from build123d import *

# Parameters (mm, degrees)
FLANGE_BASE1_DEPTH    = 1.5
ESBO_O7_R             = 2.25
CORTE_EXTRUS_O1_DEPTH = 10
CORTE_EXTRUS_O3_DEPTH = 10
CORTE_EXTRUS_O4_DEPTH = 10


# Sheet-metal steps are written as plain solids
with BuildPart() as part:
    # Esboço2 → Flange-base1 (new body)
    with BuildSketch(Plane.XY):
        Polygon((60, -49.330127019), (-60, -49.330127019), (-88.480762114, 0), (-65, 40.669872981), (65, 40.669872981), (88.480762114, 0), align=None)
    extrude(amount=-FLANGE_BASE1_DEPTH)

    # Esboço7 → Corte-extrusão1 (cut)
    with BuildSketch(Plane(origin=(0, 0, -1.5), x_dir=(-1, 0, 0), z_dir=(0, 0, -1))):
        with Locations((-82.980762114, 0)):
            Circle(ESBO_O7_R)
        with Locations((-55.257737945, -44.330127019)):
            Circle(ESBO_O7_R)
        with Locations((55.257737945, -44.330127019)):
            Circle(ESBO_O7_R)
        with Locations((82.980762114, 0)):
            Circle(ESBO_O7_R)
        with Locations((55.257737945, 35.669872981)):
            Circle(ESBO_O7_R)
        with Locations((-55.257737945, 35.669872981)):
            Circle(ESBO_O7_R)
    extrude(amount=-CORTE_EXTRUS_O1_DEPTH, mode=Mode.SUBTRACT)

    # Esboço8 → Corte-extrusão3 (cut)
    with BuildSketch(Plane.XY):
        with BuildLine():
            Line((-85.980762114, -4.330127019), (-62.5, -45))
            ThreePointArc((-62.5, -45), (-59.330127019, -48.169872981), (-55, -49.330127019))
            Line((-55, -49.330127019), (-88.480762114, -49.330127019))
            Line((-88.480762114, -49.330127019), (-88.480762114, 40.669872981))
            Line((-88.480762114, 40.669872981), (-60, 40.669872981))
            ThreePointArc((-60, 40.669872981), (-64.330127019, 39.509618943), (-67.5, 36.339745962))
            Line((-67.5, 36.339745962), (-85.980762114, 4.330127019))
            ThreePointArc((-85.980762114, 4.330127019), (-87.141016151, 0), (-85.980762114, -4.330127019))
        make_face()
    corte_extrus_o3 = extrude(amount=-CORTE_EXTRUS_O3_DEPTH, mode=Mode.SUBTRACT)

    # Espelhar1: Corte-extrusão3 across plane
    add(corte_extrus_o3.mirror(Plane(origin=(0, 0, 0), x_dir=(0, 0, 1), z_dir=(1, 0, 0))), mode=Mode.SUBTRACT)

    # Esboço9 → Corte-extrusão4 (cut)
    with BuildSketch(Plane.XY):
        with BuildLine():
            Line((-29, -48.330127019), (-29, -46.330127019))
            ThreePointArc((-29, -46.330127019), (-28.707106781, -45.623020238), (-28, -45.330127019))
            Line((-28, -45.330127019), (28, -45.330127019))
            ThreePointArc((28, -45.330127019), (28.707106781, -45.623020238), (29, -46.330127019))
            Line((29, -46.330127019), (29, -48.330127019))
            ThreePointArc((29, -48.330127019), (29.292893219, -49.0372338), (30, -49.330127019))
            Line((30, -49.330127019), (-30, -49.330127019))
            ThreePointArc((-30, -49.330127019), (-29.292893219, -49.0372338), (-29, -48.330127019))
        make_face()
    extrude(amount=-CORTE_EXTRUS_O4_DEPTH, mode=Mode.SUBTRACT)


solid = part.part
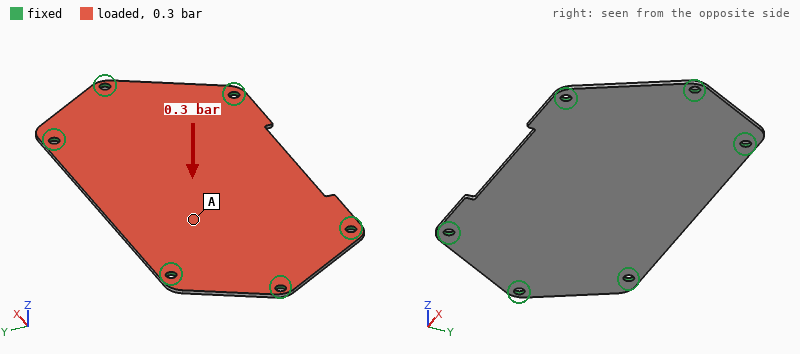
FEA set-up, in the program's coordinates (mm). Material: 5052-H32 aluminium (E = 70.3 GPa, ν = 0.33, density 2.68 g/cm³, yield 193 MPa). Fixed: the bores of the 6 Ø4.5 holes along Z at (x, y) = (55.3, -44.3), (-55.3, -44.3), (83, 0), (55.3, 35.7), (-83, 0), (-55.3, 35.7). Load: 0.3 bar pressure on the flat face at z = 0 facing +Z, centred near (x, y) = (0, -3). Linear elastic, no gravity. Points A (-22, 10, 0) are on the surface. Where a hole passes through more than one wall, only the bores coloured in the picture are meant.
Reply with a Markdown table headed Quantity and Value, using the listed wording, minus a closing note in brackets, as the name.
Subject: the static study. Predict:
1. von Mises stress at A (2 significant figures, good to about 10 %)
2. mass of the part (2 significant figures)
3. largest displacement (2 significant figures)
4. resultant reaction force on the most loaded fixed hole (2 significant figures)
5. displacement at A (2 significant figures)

| Quantity | Value |
|---|---|
| von Mises stress at A | 29 MPa |
| mass of the part | 53 g |
| largest displacement | 0.89 mm |
| resultant reaction force on the most loaded fixed hole | 91 N |
| displacement at A | 0.70 mm |
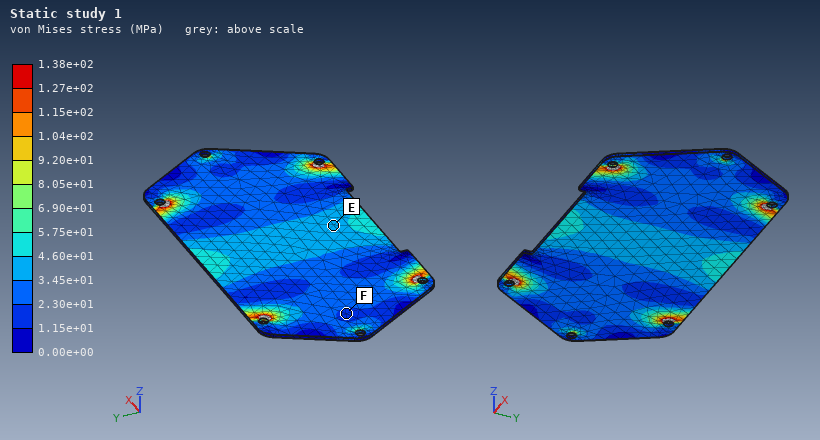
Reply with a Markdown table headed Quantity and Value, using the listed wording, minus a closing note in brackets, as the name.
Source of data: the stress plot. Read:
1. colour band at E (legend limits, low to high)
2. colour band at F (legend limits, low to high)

| Quantity | Value |
|---|---|
| colour band at E | 3.45e+01 to 4.60e+01 MPa |
| colour band at F | 1.15e+01 to 2.30e+01 MPa |
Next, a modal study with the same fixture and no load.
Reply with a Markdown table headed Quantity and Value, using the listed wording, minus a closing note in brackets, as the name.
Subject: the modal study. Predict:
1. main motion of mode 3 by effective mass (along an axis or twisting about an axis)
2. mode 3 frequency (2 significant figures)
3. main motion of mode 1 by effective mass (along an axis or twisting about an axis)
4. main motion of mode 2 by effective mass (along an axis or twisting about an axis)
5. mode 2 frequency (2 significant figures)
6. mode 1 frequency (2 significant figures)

| Quantity | Value |
|---|---|
| main motion of mode 3 by effective mass | twisting about Y |
| mode 3 frequency | 1300 Hz |
| main motion of mode 1 by effective mass | along Z |
| main motion of mode 2 by effective mass | twisting about X |
| mode 2 frequency | 880 Hz |
| mode 1 frequency | 540 Hz |
